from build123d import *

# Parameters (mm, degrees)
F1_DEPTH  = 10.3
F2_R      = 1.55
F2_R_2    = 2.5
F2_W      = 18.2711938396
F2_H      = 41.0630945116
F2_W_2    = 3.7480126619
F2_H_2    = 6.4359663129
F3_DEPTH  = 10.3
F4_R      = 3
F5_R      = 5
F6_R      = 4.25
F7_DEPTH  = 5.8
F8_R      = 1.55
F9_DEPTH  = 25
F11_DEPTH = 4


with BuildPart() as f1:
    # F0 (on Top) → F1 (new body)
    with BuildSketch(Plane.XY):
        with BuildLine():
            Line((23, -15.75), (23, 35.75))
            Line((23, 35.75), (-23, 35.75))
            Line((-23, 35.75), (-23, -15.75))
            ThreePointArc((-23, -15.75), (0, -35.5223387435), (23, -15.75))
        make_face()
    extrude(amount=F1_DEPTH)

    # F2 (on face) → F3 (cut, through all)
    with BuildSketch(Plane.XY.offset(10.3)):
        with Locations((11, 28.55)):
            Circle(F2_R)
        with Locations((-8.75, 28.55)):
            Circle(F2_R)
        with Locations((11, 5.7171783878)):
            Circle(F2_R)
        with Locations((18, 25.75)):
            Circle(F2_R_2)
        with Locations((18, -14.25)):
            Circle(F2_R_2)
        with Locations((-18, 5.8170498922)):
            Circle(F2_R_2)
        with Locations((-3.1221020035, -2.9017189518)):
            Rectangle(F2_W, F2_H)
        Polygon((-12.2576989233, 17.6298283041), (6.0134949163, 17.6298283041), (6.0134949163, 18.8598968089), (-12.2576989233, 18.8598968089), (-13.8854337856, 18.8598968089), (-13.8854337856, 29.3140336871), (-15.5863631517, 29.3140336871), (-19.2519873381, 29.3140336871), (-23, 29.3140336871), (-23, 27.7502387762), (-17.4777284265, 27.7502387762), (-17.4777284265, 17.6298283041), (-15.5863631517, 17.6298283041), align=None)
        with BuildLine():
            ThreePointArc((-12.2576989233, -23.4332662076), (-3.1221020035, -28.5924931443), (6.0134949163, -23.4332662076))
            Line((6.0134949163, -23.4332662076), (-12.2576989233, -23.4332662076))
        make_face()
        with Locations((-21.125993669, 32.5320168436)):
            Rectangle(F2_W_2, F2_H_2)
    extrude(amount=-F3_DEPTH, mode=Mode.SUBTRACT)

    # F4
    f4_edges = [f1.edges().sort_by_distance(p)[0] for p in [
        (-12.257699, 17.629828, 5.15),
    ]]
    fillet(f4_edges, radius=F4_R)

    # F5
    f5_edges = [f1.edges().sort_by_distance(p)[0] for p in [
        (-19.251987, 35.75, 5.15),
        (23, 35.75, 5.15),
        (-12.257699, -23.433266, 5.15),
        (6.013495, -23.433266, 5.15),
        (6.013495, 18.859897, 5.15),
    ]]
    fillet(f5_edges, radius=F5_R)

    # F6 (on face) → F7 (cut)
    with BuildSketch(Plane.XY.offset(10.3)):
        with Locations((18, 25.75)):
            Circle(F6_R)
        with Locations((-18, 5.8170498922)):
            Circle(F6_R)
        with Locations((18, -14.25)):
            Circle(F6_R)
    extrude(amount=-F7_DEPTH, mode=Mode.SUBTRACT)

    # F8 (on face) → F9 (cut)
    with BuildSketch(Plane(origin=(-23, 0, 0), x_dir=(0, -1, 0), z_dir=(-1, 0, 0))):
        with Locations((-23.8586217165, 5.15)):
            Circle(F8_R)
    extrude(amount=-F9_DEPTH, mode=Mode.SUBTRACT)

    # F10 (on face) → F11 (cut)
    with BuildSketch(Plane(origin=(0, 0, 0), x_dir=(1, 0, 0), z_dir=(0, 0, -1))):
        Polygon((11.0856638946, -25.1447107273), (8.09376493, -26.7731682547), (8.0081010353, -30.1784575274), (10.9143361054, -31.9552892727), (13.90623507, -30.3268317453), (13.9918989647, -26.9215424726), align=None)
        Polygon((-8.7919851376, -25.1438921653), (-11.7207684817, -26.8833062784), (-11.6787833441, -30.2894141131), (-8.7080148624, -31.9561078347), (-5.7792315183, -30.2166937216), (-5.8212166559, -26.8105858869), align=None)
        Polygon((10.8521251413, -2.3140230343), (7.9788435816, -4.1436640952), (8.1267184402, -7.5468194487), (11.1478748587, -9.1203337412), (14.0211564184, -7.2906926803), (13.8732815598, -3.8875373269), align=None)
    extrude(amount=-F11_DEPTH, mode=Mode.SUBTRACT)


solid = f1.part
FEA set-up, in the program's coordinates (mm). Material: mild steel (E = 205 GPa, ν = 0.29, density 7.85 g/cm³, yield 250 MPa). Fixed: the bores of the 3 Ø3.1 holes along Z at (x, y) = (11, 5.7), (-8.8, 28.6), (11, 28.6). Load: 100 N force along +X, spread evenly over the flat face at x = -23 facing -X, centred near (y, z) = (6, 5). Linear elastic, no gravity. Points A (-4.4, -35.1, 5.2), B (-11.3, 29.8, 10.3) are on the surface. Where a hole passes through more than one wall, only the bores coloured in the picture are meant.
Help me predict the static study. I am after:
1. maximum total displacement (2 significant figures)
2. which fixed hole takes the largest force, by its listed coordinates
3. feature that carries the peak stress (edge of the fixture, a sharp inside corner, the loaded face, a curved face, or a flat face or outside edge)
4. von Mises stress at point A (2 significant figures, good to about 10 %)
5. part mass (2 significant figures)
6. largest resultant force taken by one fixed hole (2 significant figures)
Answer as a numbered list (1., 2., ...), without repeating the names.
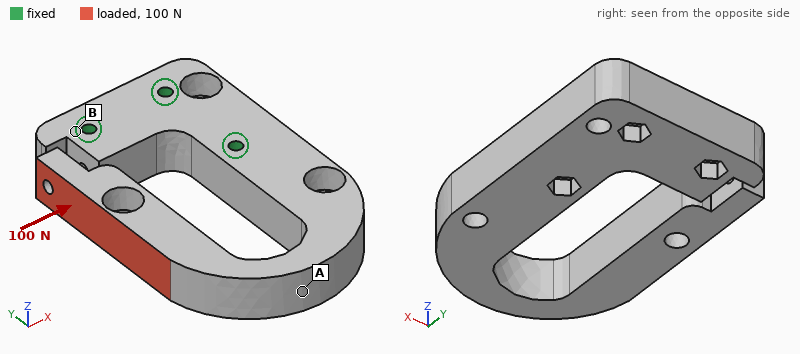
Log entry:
1. 0.13 mm
2. (11, 5.7)
3. a curved face
4. 43 MPa
5. 160 g
6. 95 N
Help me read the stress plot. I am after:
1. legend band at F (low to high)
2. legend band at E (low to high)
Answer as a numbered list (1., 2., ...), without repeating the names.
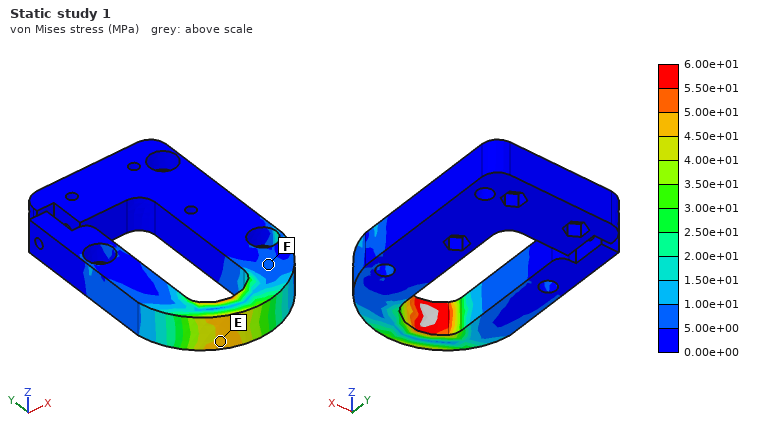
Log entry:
1. 5.00e+00 to 1.00e+01 MPa
2. 4.50e+01 to 5.00e+01 MPa
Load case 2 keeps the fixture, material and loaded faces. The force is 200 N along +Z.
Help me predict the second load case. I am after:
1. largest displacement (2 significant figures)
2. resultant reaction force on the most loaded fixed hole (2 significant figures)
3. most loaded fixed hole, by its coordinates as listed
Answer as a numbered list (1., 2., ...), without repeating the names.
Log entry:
1. 0.29 mm
2. 180 N
3. (11, 5.7)
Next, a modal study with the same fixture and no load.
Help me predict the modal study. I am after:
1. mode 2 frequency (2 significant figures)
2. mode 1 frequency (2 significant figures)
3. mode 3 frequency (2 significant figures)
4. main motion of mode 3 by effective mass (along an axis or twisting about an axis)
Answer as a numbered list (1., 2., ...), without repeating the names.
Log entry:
1. 990 Hz
2. 960 Hz
3. 2300 Hz
4. along Z
